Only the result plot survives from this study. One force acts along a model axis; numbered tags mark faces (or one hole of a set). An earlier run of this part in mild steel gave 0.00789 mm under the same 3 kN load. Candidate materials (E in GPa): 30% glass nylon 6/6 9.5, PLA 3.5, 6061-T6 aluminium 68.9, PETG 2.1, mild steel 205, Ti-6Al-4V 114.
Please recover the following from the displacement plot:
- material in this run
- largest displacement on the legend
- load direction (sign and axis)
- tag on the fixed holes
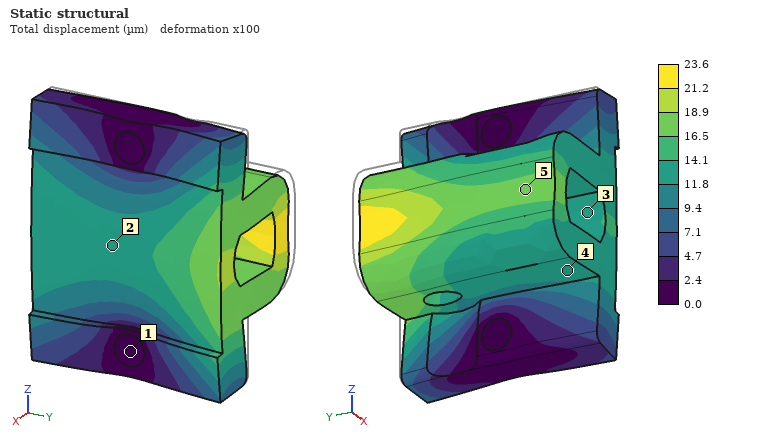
6061-T6 aluminium
23.6 µm
+X
1
